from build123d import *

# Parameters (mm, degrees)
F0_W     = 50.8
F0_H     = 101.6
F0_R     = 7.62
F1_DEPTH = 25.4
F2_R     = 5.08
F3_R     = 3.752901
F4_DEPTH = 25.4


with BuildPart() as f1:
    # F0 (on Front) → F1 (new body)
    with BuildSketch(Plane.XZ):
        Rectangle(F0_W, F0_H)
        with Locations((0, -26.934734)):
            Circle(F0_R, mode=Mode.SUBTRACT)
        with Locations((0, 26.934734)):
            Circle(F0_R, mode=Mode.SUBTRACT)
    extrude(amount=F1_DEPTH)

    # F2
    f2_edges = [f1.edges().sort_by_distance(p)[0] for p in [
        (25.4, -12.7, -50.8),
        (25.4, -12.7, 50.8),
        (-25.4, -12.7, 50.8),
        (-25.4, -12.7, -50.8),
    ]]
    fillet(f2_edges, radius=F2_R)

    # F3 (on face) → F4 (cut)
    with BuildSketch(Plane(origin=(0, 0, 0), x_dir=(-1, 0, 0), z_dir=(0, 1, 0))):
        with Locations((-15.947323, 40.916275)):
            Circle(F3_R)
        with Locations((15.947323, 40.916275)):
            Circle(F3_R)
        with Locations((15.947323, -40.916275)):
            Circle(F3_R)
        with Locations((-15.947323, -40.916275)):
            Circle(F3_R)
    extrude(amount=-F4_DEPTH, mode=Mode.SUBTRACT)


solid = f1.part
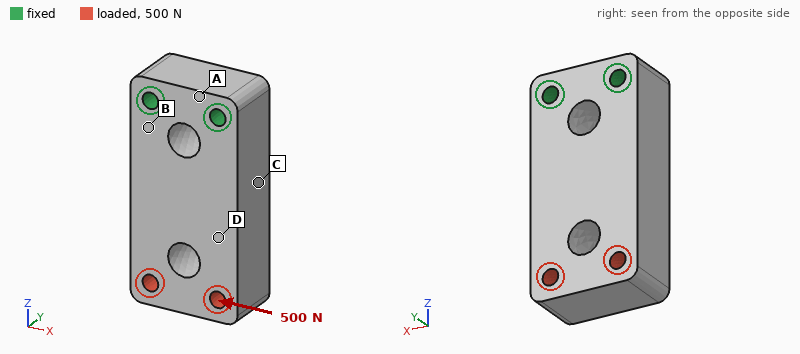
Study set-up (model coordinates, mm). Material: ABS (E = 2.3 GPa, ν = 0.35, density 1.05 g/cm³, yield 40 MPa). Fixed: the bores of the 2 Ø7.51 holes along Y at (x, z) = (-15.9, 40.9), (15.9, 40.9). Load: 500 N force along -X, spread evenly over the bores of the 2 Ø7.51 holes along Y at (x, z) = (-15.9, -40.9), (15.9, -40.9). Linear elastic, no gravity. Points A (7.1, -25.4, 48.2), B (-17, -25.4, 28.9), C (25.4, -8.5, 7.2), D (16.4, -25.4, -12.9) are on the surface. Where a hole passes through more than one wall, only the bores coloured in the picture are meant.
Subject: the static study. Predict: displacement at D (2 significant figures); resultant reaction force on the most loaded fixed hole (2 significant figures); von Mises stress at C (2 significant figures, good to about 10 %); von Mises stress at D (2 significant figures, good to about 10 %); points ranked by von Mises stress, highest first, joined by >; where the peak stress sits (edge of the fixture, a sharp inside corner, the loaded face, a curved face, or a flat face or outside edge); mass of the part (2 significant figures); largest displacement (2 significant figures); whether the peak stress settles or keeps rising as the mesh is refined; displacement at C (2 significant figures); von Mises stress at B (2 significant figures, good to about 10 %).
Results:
0.12 mm
1.1 kN
2.0 MPa
0.91 MPa
B > C > D > A
edge of the fixture
120 g
0.25 mm
keeps rising
0.081 mm
2.7 MPa
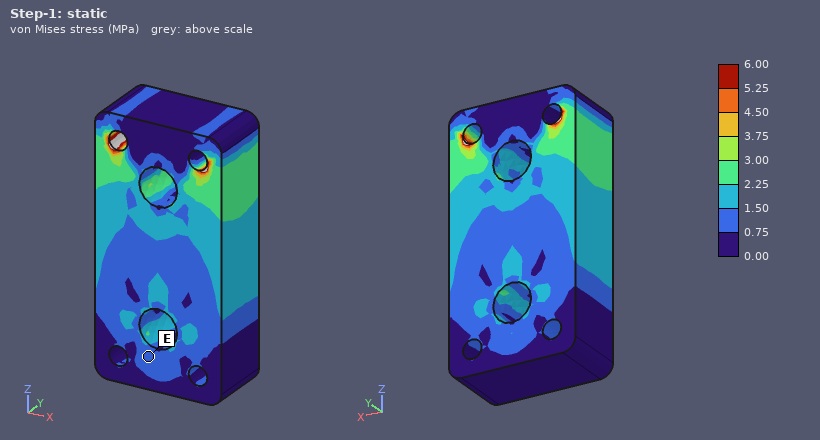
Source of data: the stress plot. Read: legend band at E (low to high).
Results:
0.75 to 1.50 MPa
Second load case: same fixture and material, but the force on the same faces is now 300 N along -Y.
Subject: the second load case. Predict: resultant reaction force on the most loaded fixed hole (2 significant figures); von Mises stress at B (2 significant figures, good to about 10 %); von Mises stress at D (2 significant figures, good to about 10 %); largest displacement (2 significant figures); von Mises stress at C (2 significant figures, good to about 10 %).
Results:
150 N
5.4 MPa
1.8 MPa
0.53 mm
1.4 MPa
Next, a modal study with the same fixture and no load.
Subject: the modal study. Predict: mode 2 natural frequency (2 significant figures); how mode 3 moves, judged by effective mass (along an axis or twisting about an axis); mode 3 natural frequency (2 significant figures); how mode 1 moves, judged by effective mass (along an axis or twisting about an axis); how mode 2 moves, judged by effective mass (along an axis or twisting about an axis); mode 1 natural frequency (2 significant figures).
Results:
1200 Hz
twisting about Z
1900 Hz
along Y
along X
660 Hz
